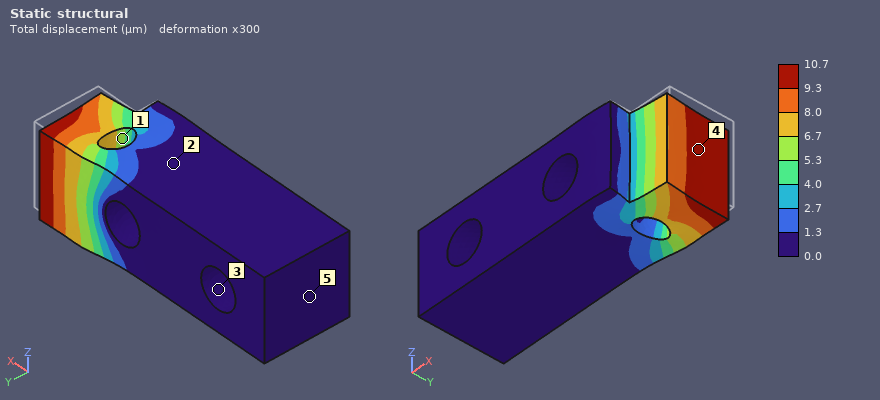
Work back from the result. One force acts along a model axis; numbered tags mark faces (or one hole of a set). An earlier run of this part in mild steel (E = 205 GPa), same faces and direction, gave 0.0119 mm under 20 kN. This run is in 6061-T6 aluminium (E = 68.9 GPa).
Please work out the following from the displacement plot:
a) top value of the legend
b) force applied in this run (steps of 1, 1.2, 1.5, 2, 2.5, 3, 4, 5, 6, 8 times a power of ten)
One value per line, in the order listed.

10.7 µm
6 kN
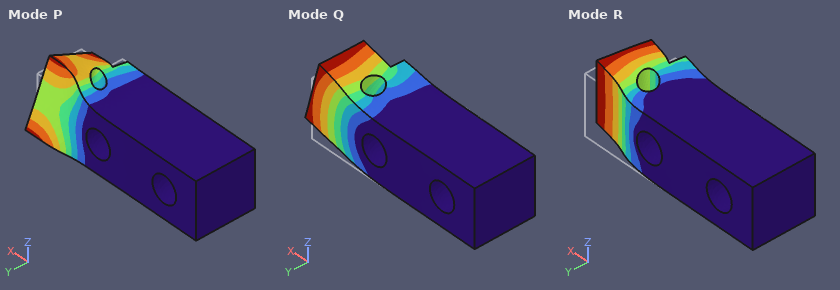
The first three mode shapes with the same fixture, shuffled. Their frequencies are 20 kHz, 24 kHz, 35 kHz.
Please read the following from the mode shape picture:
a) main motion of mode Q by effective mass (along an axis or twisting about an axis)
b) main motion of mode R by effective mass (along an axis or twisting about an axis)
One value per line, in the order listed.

along Z
along Y
